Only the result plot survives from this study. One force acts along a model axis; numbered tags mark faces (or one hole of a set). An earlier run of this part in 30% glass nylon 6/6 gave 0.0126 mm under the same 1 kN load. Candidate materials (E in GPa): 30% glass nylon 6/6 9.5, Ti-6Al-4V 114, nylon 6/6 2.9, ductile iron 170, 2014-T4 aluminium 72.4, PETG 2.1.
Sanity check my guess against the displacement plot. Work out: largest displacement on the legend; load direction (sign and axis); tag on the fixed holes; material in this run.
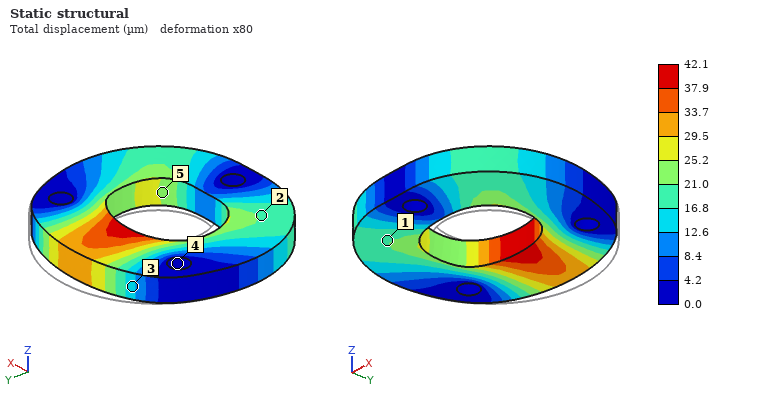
42.1 µm
-Y
4
nylon 6/6
